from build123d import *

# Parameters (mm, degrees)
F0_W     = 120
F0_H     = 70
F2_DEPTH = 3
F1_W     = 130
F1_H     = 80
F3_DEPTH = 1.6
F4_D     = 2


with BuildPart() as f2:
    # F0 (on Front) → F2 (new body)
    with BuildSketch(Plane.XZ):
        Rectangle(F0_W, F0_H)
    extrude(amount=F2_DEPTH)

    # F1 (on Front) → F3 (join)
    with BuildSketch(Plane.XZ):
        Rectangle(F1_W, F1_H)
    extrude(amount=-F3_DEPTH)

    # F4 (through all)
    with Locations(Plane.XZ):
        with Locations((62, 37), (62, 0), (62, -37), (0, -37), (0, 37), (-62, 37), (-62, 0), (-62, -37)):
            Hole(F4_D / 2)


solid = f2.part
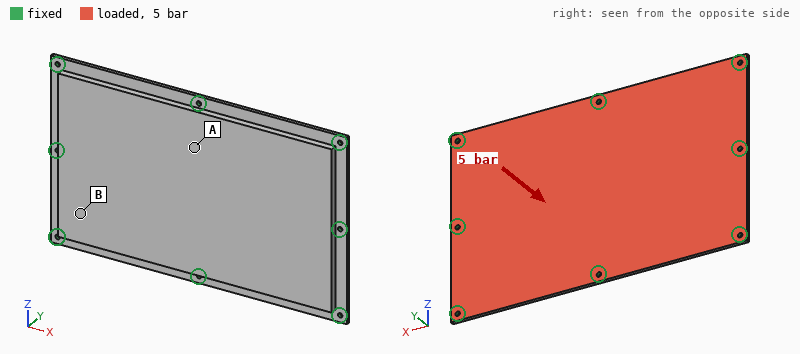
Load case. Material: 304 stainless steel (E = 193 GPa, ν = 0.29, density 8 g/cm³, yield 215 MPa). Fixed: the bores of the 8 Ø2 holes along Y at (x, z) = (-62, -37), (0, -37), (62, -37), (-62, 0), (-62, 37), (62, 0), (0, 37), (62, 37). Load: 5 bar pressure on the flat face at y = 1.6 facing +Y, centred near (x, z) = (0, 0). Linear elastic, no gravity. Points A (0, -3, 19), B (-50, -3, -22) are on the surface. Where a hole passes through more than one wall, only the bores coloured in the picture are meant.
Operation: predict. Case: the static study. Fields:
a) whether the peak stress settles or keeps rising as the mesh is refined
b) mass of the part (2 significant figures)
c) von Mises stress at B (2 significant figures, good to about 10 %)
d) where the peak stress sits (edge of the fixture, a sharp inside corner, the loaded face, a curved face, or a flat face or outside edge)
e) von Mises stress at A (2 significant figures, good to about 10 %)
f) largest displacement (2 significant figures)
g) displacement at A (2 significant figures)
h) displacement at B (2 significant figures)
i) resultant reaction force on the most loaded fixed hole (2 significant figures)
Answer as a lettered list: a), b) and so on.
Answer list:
a) keeps rising
b) 330 g
c) 23 MPa
d) edge of the fixture
e) 60 MPa
f) 78 µm
g) 56 µm
h) 31 µm
i) 2.3 kN
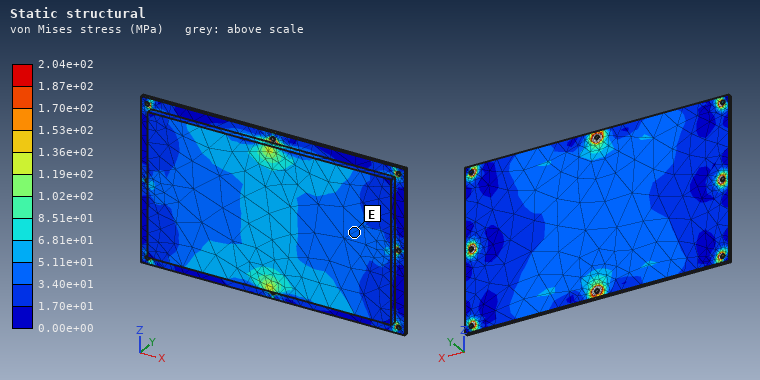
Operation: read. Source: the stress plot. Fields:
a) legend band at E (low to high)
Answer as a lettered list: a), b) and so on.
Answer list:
a) 3.40e+01 to 5.11e+01 MPa
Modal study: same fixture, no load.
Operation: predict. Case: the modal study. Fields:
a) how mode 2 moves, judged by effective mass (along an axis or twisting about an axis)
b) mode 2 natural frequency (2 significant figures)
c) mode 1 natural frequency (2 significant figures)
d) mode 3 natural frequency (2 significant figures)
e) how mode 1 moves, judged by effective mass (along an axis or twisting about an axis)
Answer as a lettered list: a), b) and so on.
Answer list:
a) twisting about Z
b) 3100 Hz
c) 2500 Hz
d) 4200 Hz
e) along Y
